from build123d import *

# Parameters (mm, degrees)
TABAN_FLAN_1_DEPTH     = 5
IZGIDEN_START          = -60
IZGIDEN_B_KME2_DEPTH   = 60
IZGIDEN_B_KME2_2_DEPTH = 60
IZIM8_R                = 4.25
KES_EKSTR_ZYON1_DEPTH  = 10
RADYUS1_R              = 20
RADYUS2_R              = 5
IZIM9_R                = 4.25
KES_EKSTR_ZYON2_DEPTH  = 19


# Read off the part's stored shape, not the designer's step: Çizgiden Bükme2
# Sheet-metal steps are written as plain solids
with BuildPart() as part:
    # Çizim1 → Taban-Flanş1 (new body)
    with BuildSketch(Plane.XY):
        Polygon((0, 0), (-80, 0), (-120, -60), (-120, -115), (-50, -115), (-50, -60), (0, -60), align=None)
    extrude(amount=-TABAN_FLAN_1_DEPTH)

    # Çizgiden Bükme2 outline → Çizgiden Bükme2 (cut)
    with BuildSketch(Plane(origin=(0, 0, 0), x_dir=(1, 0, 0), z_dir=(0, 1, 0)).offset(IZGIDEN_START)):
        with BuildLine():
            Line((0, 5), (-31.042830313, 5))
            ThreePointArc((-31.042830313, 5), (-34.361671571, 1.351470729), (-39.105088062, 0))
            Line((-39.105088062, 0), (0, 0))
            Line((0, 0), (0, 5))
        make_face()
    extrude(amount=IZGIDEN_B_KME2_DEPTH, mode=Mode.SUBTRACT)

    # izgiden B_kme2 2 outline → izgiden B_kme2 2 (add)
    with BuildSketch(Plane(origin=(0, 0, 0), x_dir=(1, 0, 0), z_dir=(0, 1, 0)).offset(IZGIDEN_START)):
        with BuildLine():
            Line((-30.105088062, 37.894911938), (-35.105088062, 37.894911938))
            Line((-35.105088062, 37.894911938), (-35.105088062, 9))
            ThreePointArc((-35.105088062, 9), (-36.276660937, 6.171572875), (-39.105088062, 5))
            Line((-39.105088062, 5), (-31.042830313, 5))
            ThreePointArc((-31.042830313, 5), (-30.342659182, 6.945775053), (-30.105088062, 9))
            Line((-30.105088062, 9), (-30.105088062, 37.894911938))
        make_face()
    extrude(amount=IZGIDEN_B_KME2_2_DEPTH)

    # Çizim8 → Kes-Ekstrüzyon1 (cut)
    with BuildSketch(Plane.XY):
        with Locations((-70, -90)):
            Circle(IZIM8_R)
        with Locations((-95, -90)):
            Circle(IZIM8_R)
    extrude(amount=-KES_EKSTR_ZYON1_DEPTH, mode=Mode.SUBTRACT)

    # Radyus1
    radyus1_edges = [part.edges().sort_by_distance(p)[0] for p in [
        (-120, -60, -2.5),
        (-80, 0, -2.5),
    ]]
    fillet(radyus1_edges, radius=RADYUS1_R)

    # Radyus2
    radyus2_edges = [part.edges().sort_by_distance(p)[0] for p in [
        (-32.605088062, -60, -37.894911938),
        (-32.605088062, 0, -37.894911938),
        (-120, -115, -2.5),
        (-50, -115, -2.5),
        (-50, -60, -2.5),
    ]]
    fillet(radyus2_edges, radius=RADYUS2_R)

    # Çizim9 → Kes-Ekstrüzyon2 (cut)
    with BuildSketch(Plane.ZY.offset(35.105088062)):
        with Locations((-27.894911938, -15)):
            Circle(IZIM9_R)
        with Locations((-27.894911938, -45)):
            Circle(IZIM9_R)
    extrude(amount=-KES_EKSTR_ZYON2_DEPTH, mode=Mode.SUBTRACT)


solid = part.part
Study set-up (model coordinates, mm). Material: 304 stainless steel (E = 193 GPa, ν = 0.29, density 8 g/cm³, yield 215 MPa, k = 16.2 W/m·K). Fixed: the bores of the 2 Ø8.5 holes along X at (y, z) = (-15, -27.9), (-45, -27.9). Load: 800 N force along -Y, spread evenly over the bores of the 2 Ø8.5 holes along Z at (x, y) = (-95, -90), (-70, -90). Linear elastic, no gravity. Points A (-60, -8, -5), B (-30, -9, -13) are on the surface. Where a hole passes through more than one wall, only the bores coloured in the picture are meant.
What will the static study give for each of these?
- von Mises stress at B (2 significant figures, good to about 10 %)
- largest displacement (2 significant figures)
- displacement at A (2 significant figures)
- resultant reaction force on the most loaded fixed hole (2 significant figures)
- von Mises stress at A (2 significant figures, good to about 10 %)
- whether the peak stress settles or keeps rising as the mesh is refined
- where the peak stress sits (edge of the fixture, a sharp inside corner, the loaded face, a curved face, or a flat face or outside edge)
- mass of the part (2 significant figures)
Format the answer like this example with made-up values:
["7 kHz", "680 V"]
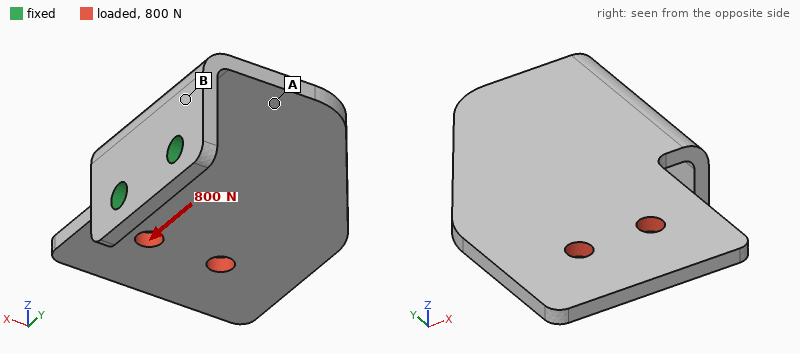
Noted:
["44 MPa", "0.25 mm", "0.072 mm", "1.2 kN", "19 MPa", "keeps rising", "edge of the fixture", "380 g"]
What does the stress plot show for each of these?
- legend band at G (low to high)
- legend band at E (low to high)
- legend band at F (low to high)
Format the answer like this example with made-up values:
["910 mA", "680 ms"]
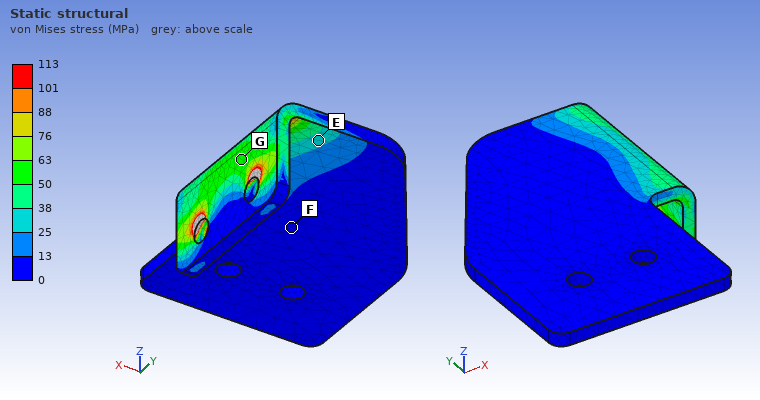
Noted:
["50 to 63 MPa", "25 to 38 MPa", "0 to 13 MPa"]
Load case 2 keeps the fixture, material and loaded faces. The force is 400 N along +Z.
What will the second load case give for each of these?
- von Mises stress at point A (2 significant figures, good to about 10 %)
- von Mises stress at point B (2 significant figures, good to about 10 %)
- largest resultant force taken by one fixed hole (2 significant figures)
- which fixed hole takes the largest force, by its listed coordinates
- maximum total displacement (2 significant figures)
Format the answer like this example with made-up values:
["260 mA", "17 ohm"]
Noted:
["54 MPa", "52 MPa", "860 N", "(-45, -27.9)", "1.1 mm"]
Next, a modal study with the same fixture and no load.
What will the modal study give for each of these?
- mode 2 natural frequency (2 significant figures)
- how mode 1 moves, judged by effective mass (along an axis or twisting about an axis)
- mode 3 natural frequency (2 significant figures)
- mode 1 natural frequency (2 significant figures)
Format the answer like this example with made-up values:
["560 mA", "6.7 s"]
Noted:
["630 Hz", "along Z", "790 Hz", "280 Hz"]
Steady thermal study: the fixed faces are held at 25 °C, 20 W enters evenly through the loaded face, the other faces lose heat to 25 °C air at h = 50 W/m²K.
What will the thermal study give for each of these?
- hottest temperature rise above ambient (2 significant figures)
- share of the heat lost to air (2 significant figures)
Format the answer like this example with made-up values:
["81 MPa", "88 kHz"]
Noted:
["71 K", "98 %"]
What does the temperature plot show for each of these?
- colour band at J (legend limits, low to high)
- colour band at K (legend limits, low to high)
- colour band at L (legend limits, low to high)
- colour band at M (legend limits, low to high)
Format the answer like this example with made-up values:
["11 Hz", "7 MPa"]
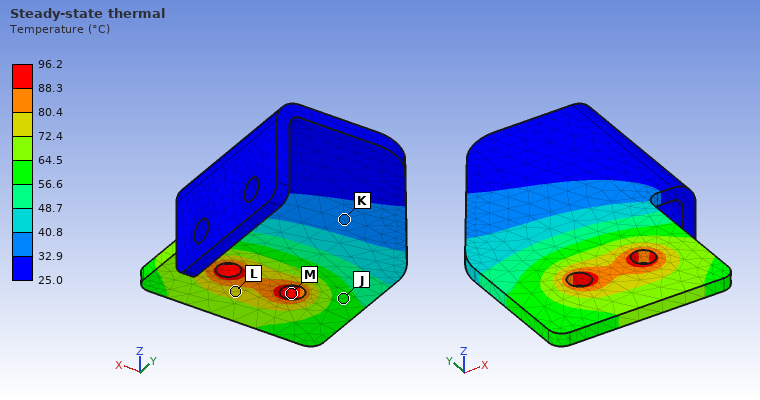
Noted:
["56.6 to 64.5 °C", "32.9 to 40.8 °C", "72.4 to 80.4 °C", "88.3 to 96.2 °C"]
